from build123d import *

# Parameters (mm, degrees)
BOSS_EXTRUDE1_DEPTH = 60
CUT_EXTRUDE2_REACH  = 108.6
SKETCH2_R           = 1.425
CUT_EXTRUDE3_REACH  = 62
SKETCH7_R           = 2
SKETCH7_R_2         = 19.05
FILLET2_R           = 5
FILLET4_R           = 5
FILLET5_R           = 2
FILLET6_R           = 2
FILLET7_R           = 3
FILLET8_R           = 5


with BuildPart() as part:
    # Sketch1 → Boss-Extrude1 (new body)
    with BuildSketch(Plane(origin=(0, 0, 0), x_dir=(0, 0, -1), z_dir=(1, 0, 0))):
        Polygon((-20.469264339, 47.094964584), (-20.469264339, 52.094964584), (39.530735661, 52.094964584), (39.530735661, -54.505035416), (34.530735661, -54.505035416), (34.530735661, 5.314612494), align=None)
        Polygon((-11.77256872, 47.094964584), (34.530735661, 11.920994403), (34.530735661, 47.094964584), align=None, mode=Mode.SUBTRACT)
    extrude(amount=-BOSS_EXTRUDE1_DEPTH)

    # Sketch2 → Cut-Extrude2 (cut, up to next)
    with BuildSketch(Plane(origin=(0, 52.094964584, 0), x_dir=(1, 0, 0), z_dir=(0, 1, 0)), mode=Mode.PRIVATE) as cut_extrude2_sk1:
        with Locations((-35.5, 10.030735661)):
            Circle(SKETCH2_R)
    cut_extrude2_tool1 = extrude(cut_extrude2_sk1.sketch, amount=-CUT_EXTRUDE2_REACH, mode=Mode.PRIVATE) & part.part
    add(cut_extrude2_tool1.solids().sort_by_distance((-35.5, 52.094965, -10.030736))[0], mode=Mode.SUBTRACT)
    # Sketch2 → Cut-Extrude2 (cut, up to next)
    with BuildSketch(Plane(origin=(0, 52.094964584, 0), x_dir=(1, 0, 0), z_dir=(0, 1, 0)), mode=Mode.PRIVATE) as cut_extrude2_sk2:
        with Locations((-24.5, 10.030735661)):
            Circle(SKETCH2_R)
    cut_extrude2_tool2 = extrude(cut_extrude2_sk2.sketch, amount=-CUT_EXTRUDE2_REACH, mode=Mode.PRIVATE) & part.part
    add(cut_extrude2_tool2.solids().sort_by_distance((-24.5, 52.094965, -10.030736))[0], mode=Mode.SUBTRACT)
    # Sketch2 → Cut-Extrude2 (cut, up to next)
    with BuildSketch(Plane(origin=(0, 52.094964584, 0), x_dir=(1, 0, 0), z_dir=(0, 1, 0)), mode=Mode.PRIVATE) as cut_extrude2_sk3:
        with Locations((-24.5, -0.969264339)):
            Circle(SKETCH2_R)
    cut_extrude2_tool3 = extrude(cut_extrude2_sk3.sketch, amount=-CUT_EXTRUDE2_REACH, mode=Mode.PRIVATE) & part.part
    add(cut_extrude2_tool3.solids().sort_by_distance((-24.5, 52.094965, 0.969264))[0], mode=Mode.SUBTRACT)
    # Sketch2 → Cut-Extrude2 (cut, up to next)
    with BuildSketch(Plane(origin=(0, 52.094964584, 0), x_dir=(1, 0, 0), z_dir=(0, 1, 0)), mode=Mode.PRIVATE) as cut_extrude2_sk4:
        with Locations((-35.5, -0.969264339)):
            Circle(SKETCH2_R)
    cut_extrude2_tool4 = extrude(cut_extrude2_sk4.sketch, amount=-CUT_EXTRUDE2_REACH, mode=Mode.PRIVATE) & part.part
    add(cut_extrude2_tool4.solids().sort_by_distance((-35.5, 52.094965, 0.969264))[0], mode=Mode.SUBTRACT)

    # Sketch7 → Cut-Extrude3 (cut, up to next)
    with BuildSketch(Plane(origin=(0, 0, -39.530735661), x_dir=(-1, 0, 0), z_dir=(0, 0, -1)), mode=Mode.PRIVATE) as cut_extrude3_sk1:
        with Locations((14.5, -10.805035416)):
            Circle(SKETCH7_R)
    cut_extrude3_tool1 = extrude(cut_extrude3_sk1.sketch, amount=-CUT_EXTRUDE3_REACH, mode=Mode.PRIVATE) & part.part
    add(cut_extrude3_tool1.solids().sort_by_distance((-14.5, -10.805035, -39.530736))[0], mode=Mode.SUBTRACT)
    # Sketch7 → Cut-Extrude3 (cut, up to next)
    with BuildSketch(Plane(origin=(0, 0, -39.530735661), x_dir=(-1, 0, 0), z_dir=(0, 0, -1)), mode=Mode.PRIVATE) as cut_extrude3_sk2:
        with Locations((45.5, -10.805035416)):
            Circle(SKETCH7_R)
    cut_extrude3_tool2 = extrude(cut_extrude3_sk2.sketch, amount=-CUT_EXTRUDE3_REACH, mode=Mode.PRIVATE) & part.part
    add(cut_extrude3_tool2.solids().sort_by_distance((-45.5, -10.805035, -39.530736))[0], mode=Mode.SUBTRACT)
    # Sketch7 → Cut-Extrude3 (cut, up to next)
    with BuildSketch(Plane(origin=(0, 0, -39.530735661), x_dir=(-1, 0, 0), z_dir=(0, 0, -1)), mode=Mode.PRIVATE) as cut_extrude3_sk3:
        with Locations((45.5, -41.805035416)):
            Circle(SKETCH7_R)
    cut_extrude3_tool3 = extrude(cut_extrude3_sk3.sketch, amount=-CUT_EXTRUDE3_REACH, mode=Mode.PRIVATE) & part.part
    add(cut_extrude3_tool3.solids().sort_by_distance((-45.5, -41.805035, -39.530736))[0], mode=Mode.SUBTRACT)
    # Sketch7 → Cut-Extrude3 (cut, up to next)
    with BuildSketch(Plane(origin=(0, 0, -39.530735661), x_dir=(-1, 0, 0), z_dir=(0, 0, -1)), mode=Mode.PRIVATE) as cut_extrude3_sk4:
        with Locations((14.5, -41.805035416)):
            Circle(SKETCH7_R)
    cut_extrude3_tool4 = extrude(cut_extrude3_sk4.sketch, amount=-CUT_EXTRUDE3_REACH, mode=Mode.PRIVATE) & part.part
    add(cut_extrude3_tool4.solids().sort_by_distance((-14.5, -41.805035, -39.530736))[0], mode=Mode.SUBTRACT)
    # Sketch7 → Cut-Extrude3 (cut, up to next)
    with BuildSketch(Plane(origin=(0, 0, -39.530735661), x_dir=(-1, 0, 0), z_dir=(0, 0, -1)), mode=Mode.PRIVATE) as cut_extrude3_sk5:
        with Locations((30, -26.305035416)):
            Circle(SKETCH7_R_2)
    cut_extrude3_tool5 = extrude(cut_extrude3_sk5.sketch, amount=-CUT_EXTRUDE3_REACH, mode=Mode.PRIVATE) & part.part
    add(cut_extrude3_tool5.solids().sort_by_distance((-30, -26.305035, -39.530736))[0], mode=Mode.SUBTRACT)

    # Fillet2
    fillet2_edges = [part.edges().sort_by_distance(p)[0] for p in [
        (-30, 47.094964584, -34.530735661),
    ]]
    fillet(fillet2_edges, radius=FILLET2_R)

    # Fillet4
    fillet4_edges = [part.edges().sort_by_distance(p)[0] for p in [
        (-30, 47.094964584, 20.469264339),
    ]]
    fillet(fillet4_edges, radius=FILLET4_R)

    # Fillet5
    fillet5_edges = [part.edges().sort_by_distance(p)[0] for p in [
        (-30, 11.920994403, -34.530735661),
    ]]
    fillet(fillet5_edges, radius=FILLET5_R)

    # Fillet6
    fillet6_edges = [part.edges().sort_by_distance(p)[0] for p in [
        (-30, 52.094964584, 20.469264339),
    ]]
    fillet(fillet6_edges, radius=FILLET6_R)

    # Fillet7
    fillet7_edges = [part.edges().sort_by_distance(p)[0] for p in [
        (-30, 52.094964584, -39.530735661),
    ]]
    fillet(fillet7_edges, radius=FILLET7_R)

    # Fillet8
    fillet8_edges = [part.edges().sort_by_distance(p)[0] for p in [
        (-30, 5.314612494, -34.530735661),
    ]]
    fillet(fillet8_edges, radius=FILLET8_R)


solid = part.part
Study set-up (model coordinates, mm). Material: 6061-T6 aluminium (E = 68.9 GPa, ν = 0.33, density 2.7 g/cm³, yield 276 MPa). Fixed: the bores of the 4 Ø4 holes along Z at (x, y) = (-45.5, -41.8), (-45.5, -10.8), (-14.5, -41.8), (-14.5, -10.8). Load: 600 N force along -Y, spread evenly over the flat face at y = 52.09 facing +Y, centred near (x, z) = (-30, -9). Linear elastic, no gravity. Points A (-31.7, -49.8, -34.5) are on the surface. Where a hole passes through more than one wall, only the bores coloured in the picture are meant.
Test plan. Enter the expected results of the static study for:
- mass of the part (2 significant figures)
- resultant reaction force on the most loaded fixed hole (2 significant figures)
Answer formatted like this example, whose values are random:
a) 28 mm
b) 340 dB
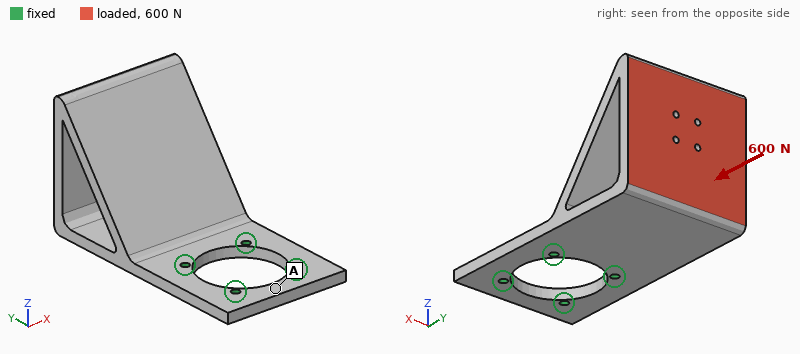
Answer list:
a) 170 g
b) 290 N
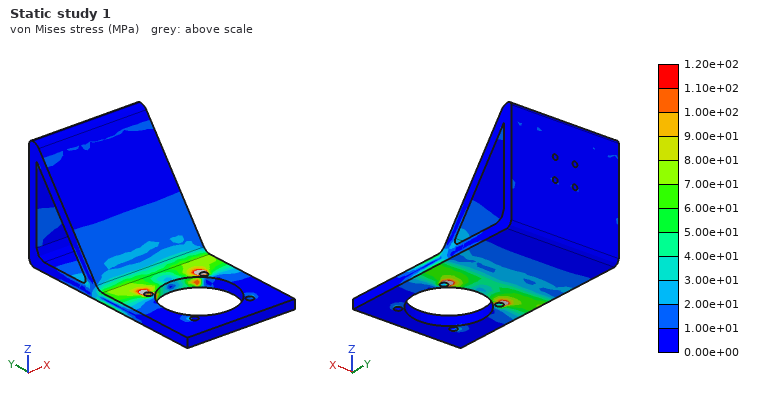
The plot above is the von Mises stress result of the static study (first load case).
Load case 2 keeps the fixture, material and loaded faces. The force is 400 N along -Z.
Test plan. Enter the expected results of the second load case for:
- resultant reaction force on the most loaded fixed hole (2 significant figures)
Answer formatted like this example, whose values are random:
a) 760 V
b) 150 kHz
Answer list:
a) 280 N
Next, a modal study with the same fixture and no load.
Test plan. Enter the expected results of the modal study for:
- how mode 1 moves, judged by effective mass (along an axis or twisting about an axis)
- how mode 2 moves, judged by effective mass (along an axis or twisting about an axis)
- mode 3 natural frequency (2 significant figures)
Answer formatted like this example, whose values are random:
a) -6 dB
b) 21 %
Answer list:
a) along Z
b) along X
c) 3300 Hz
